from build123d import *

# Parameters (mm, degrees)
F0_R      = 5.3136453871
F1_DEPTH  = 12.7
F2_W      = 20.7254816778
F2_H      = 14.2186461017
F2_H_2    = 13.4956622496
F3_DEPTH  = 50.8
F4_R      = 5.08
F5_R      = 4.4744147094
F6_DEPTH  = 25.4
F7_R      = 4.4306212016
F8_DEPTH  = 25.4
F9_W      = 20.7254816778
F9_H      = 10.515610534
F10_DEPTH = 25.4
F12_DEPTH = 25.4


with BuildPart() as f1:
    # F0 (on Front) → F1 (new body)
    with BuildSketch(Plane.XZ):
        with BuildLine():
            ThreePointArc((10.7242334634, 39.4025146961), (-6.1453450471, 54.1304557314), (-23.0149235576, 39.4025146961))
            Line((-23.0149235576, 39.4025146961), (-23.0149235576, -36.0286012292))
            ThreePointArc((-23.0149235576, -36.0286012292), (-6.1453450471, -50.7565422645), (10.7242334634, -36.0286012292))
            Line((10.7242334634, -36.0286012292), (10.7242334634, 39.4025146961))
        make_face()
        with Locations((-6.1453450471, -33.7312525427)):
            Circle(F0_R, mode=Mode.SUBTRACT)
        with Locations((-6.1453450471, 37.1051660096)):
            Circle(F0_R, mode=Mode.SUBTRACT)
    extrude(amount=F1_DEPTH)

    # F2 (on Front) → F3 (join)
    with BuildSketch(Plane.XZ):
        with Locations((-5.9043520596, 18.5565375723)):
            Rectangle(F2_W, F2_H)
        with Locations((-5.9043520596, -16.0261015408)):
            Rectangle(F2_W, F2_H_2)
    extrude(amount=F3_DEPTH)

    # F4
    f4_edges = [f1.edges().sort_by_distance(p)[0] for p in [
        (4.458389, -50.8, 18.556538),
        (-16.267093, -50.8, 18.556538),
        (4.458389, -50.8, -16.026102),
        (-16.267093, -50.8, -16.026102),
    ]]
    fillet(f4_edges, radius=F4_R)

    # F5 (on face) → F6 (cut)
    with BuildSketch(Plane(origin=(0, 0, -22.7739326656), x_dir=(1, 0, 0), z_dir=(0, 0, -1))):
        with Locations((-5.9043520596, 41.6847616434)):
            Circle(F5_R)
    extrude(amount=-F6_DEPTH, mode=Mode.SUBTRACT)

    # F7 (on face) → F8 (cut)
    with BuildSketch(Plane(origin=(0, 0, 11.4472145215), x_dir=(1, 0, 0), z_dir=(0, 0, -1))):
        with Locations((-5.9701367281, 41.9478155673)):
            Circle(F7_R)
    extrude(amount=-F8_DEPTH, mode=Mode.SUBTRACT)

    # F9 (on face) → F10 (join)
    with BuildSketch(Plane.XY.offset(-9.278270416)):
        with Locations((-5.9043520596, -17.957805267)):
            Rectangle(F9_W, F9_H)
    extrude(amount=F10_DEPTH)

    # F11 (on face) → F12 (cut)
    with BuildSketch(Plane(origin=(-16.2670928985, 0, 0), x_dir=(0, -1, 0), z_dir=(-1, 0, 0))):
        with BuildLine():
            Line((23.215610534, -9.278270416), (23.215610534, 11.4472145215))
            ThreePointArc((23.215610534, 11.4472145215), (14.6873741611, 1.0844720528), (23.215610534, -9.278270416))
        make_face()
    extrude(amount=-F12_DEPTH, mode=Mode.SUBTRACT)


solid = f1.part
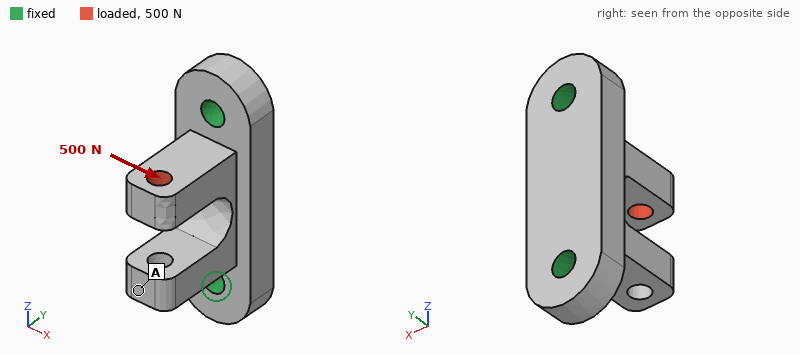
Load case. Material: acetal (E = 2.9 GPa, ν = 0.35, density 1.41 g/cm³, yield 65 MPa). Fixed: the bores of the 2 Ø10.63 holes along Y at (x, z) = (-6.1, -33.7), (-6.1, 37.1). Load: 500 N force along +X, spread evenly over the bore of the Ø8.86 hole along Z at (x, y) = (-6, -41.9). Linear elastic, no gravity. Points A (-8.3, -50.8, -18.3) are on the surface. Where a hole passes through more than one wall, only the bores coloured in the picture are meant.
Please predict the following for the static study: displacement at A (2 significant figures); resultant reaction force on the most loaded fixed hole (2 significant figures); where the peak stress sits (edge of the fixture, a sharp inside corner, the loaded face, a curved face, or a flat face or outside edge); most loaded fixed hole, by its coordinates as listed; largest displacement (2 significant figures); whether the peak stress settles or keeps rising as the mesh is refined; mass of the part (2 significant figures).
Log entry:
0.17 mm
390 N
edge of the fixture
(-6.1, 37.1)
0.62 mm
keeps rising
86 g
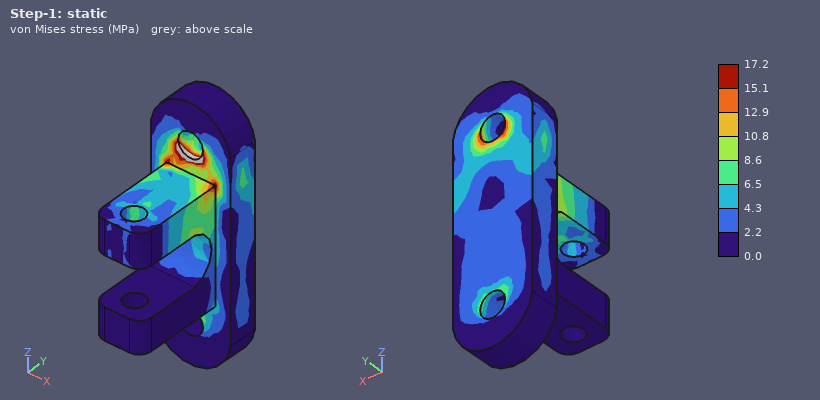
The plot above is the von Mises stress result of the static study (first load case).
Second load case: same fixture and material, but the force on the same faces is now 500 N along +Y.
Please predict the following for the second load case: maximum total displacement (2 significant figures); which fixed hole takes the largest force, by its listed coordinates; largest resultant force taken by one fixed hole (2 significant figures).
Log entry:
58 µm
(-6.1, 37.1)
410 N
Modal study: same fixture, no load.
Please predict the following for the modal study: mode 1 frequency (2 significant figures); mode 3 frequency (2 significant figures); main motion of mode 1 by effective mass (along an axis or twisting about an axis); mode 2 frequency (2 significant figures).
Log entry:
1600 Hz
2200 Hz
along X
1800 Hz
